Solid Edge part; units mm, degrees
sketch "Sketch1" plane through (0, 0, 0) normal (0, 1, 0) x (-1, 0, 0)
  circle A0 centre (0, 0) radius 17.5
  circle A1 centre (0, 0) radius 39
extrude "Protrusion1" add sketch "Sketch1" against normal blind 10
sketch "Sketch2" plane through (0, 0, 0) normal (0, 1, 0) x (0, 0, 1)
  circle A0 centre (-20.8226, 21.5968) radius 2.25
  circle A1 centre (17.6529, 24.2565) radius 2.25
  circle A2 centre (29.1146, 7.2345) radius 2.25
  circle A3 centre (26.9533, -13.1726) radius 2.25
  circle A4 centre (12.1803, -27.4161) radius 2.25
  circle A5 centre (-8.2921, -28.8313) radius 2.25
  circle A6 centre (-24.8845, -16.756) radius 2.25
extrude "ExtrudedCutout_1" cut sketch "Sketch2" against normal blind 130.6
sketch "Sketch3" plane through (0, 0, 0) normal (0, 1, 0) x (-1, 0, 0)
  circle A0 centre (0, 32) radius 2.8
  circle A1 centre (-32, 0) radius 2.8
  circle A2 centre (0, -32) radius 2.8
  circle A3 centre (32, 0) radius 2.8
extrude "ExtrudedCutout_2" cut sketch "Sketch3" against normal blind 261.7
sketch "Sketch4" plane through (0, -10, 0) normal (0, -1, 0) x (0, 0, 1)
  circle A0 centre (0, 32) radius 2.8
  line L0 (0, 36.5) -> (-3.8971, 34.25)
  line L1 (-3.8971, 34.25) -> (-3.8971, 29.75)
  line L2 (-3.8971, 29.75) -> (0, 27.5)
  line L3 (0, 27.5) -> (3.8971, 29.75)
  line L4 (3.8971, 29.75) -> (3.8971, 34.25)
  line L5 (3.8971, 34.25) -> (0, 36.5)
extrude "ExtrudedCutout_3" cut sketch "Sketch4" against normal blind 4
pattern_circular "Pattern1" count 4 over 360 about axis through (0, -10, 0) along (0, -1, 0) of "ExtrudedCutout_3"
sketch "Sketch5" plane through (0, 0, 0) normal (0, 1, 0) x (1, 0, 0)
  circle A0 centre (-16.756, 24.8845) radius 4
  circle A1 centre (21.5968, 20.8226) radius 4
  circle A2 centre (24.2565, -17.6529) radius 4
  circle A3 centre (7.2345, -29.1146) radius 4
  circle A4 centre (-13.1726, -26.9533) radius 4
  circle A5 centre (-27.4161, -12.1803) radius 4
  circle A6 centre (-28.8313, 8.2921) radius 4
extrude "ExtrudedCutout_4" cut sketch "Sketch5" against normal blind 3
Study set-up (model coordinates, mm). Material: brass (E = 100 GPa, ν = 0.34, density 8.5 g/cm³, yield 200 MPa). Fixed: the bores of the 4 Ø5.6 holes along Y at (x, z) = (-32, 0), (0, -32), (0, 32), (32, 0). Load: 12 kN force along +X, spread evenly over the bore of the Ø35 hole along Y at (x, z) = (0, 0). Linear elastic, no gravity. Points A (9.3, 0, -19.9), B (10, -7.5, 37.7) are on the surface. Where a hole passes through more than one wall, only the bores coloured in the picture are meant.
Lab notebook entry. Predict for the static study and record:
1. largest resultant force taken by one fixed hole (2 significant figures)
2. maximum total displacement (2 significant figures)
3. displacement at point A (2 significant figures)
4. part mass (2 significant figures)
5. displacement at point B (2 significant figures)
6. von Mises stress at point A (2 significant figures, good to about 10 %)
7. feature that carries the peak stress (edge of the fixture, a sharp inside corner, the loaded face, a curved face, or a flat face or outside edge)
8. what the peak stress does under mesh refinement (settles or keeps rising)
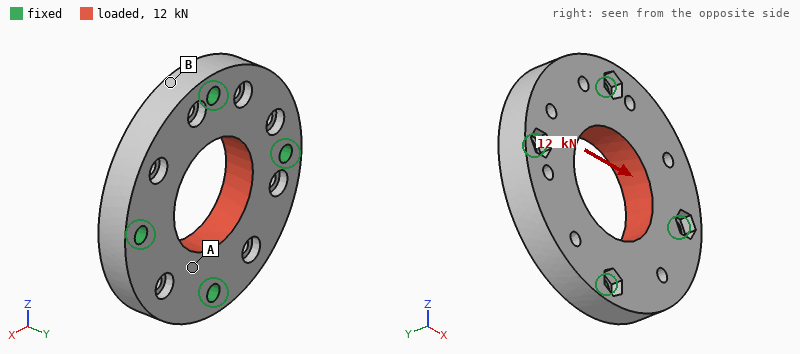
3.3 kN
6.4 µm
4.2 µm
300 g
2.2 µm
13 MPa
edge of the fixture
keeps rising
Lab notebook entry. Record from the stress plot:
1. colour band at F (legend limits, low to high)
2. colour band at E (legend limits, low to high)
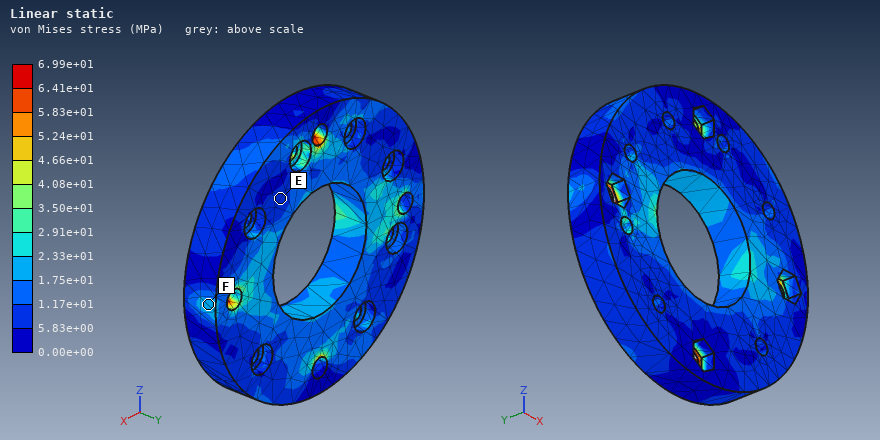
1.75e+01 to 2.33e+01 MPa
5.83e+00 to 1.17e+01 MPa
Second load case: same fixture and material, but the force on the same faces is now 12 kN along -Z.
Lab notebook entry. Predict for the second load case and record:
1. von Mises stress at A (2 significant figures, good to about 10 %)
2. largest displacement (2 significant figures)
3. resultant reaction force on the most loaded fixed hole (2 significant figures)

18 MPa
6.3 µm
3.3 kN
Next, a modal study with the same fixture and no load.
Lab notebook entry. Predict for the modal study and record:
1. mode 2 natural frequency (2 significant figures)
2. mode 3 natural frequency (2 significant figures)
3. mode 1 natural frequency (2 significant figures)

9000 Hz
9400 Hz
7900 Hz
